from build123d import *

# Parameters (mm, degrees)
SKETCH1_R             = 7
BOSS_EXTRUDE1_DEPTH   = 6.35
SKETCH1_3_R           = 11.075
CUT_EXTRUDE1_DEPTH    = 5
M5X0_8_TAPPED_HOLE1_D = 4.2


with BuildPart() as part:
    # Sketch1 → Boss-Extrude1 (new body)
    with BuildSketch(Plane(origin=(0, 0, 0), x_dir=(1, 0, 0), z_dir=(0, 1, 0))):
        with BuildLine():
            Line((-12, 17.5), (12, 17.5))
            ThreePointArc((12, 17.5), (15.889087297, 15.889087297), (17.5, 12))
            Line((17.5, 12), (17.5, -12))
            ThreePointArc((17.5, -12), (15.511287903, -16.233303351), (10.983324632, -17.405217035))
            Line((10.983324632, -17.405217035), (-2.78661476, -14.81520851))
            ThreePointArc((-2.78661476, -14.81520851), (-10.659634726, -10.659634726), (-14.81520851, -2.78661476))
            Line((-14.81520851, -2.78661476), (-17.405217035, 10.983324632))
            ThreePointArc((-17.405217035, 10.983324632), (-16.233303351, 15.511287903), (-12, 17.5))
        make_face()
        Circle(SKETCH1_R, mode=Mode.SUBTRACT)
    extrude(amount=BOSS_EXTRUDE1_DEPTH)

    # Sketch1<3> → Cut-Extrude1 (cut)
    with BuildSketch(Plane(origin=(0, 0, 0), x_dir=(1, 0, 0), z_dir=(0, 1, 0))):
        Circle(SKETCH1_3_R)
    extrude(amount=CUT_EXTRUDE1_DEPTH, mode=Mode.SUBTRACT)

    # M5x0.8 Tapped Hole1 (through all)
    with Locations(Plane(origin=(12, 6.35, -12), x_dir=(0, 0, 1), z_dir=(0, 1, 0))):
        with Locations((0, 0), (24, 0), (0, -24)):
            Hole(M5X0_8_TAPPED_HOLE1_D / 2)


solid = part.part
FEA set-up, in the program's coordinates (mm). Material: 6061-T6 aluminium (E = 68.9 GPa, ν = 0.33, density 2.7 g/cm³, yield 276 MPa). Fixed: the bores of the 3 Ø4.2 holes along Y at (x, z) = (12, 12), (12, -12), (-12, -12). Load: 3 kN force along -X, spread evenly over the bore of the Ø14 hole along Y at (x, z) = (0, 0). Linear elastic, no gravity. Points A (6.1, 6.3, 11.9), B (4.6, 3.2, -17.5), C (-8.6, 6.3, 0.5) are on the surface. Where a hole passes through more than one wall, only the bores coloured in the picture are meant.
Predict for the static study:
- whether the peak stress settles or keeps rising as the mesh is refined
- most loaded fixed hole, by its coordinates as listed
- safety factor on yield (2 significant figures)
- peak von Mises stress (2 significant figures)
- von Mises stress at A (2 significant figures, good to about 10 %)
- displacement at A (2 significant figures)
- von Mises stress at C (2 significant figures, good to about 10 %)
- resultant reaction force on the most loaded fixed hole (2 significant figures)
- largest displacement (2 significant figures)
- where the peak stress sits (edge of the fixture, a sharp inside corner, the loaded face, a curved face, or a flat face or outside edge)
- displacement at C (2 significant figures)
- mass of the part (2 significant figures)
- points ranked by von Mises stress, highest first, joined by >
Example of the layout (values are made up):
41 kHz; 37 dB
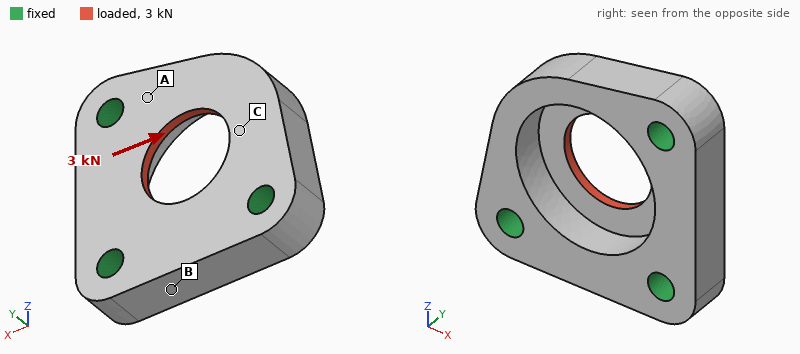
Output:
settles; (12, 12); 2.5; 110 MPa; 36 MPa; 2.9 µm; 58 MPa; 1.4 kN; 19 µm; the loaded face; 16 µm; 12 g; C > A > B
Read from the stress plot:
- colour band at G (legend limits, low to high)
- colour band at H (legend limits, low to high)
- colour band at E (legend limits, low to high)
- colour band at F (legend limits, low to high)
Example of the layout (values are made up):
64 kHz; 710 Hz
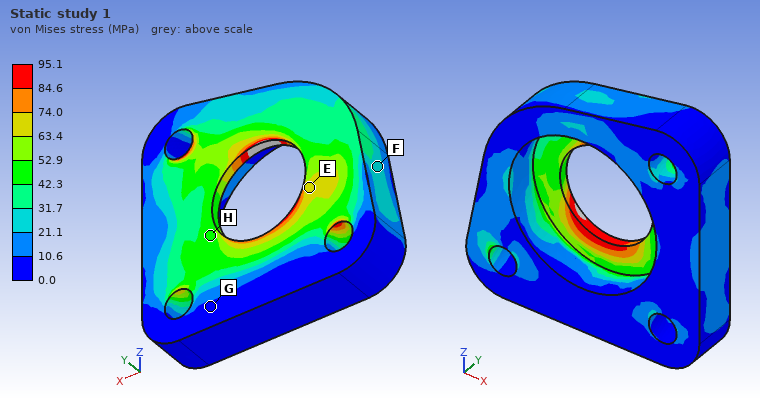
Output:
0.0 to 10.6 MPa; 42.3 to 52.9 MPa; 63.4 to 74.0 MPa; 21.1 to 31.7 MPa
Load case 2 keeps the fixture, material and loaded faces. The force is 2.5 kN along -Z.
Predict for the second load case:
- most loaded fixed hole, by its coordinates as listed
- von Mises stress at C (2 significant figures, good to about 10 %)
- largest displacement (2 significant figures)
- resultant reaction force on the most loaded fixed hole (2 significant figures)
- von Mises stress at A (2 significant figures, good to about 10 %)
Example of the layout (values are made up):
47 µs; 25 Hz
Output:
(-12, -12); 46 MPa; 16 µm; 1.1 kN; 45 MPa
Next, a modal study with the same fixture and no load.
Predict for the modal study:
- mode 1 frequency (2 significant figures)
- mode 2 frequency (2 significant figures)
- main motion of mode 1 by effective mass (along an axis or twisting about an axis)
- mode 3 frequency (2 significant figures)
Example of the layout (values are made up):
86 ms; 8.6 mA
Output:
17 kHz; 35 kHz; along Y; 42 kHz
